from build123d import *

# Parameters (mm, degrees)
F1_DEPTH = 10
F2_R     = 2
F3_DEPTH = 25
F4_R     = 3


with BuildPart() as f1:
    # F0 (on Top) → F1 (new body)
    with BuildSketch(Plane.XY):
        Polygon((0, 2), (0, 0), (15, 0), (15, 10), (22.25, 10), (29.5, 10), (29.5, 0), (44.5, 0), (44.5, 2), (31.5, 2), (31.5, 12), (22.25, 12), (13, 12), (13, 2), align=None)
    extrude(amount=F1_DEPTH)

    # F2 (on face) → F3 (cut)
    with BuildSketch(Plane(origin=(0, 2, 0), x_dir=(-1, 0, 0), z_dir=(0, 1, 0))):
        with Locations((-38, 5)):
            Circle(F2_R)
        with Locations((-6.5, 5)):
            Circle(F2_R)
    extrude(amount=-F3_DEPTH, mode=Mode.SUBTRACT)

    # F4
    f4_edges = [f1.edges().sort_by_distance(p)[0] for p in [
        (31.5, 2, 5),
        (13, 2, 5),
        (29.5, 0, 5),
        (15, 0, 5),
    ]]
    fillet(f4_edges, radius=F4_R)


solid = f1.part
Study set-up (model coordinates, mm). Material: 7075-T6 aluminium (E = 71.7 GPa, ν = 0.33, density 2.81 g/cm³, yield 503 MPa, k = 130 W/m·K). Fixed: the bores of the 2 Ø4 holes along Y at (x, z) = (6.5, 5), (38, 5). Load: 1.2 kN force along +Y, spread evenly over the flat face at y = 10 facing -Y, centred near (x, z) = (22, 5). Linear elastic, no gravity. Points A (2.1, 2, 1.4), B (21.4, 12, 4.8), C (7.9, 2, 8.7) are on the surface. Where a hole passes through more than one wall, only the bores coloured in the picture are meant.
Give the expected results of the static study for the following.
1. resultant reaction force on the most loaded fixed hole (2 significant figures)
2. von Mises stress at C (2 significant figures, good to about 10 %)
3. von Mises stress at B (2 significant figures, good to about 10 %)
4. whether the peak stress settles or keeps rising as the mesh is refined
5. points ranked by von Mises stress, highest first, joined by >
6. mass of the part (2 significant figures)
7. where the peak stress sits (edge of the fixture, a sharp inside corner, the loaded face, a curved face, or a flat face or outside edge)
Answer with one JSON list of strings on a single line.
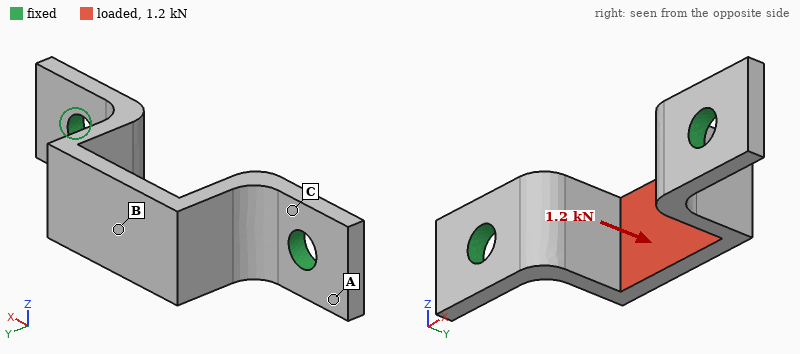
["710 N", "73 MPa", "160 MPa", "keeps rising", "B > C > A", "3.5 g", "edge of the fixture"]
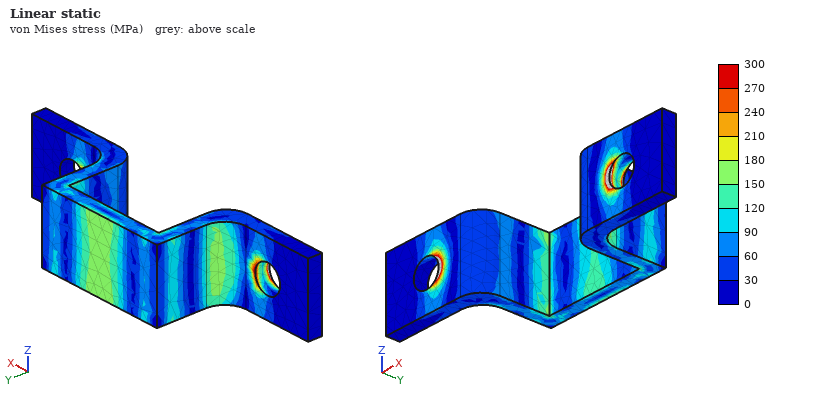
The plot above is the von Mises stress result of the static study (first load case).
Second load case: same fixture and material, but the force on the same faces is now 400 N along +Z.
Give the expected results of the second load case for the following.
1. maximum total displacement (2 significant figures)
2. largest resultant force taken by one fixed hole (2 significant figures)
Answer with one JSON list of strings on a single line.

["0.11 mm", "200 N"]
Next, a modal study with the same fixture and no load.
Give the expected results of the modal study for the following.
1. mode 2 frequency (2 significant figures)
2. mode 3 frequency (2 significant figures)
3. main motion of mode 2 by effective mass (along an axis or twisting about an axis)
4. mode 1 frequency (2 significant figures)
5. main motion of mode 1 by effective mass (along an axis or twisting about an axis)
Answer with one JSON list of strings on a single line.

["11 kHz", "14 kHz", "along X", "8100 Hz", "along Z"]
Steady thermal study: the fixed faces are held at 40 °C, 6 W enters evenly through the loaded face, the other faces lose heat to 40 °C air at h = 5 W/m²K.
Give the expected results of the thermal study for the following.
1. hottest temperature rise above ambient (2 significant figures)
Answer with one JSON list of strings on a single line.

["21 K"]
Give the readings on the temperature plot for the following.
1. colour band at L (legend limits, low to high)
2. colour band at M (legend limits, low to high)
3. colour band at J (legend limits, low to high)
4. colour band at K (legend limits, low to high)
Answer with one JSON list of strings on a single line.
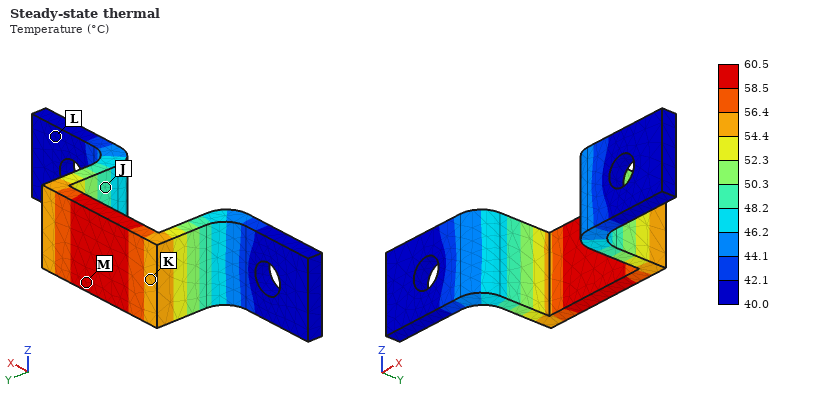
["40.0 to 42.1 °C", "58.5 to 60.5 °C", "48.2 to 50.3 °C", "54.4 to 56.4 °C"]
